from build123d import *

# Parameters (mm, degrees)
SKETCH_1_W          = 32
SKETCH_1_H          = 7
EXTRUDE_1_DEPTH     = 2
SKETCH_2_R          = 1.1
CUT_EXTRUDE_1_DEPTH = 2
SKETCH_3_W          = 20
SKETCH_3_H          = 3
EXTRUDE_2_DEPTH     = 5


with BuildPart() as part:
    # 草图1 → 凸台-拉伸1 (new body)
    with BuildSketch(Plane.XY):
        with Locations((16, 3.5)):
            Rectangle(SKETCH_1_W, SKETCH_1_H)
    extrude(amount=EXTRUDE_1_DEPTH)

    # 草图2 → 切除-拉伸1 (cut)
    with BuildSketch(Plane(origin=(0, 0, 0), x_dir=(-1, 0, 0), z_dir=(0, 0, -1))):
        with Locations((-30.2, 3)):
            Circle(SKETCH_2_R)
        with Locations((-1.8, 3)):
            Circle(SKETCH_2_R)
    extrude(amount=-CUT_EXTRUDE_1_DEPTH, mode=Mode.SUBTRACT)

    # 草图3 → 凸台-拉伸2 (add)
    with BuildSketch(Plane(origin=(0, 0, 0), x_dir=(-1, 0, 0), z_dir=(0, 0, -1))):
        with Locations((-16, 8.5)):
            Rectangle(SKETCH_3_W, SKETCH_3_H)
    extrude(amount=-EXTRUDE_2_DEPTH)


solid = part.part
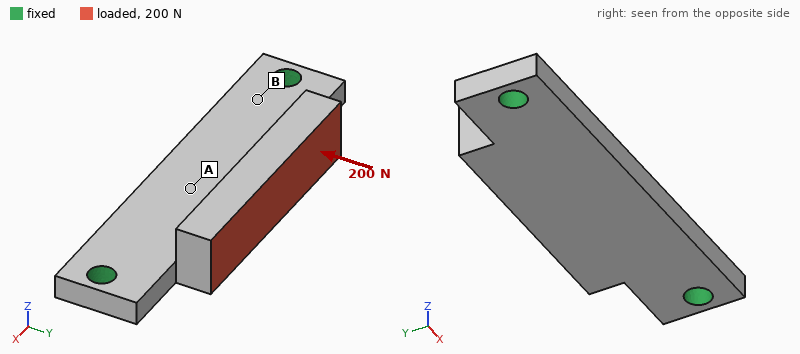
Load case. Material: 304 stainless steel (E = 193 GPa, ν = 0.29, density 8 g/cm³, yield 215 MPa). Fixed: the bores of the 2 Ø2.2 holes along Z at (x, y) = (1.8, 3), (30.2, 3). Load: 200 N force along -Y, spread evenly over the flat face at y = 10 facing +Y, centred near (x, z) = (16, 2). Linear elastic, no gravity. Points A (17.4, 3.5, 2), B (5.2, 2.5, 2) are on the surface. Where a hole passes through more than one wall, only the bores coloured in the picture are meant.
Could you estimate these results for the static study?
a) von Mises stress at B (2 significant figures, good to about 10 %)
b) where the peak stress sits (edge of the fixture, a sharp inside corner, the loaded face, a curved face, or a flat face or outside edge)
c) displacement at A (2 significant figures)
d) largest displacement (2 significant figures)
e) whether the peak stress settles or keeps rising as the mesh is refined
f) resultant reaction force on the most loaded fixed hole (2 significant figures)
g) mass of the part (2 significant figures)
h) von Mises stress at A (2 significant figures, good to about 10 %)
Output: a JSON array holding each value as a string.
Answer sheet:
["38 MPa", "edge of the fixture", "2.7 µm", "9.2 µm", "keeps rising", "120 N", "5.9 g", "8.4 MPa"]
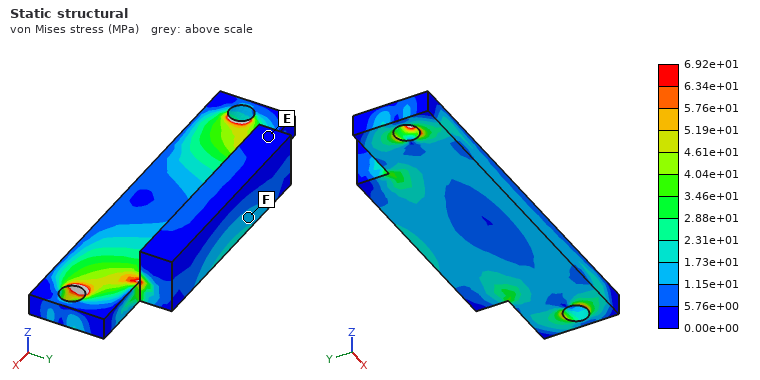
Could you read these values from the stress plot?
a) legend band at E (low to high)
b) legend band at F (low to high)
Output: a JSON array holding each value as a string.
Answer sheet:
["0.00e+00 to 5.76e+00 MPa", "1.15e+01 to 1.73e+01 MPa"]
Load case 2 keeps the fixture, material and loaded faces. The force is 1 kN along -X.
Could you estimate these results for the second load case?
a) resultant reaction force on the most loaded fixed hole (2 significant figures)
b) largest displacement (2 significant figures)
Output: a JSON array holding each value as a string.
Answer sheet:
["570 N", "5.9 µm"]
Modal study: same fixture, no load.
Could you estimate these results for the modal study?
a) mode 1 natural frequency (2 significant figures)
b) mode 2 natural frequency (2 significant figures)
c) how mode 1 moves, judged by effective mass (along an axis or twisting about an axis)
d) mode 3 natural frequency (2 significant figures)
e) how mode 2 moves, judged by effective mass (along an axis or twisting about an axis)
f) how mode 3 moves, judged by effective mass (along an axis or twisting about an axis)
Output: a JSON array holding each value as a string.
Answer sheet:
["9900 Hz", "17 kHz", "along Z", "26 kHz", "along Z", "twisting about Y"]
